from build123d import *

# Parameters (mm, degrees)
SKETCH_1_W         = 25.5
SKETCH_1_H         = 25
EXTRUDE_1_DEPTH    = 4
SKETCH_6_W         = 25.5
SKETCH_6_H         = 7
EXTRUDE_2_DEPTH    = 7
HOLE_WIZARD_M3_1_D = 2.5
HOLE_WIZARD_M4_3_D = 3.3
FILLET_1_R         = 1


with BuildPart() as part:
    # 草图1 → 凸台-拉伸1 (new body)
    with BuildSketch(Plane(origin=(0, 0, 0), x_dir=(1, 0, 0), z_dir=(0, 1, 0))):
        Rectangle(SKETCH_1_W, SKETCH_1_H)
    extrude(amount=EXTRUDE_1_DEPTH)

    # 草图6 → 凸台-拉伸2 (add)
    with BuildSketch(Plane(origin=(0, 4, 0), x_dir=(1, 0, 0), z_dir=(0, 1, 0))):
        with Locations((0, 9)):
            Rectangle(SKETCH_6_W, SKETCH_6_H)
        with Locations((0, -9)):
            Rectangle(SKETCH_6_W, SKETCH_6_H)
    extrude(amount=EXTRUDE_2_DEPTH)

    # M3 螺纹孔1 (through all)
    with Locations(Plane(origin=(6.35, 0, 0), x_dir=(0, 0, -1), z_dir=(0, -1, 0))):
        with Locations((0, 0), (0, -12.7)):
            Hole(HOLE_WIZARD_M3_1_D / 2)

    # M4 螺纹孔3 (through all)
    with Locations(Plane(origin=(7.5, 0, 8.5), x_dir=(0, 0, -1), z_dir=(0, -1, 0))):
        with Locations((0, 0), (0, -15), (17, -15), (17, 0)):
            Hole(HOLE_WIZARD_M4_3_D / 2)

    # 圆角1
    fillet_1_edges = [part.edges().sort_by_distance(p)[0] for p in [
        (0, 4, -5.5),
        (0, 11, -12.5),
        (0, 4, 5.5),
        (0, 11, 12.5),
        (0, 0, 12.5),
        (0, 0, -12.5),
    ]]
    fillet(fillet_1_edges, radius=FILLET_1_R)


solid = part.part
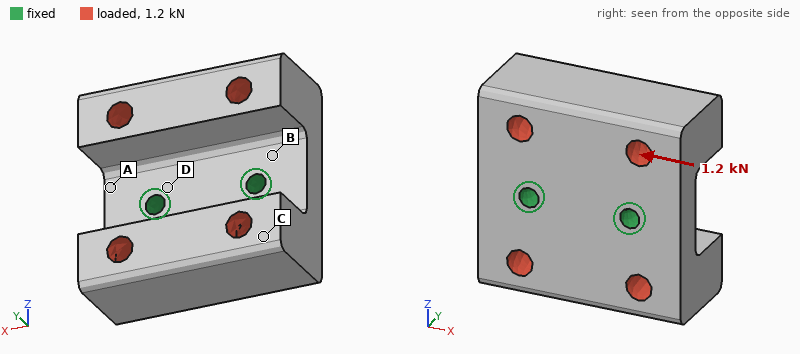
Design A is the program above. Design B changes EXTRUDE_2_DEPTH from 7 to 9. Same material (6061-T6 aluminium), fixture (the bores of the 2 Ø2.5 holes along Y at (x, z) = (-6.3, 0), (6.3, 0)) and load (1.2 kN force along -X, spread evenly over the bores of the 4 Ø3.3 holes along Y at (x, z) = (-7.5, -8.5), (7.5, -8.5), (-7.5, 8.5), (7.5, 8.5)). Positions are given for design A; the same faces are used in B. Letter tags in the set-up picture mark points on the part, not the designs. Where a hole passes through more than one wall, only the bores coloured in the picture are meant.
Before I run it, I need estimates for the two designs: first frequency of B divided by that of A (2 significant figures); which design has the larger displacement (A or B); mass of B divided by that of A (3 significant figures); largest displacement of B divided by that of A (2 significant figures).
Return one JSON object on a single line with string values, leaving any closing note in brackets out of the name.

{"first frequency of B divided by that of A": "0.85", "which design has the larger displacement": "B", "mass of B divided by that of A": "1.14", "largest displacement of B divided by that of A": "1.3"}
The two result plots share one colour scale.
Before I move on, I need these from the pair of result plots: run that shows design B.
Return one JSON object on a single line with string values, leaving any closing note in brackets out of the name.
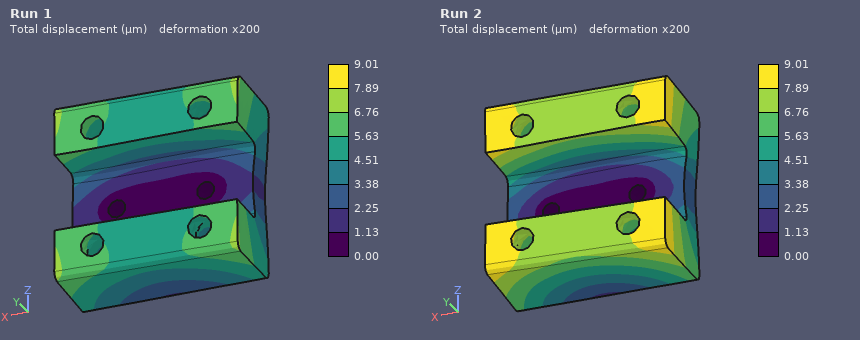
{"run that shows design B": "Run 2"}
